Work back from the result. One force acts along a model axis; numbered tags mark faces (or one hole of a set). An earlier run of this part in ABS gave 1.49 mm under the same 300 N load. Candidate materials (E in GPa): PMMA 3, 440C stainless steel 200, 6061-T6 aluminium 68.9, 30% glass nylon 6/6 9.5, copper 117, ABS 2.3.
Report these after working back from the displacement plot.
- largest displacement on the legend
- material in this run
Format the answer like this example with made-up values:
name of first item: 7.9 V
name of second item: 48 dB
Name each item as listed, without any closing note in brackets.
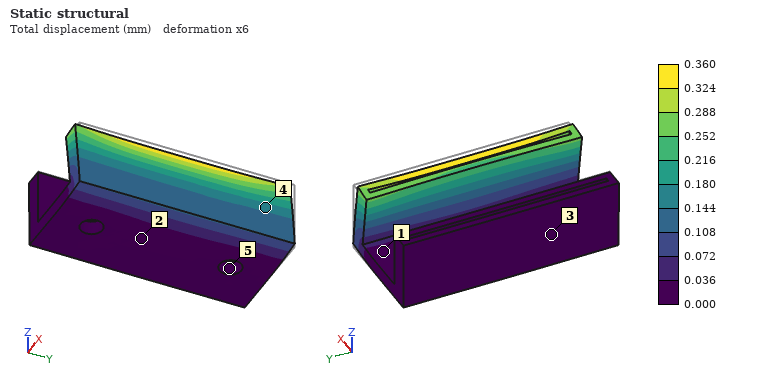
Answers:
largest displacement on the legend: 0.360 mm
material in this run: 30% glass nylon 6/6
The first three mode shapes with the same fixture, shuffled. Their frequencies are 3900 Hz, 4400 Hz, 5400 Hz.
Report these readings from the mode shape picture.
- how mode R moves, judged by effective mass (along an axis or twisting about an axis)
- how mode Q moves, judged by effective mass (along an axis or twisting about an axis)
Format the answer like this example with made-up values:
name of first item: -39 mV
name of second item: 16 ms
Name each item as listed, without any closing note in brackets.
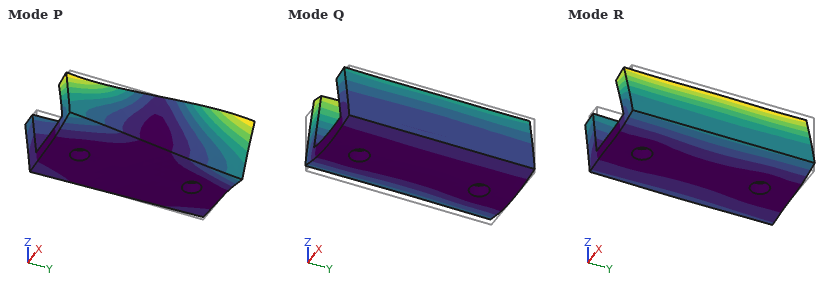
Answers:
how mode R moves, judged by effective mass: along X
how mode Q moves, judged by effective mass: along Z
